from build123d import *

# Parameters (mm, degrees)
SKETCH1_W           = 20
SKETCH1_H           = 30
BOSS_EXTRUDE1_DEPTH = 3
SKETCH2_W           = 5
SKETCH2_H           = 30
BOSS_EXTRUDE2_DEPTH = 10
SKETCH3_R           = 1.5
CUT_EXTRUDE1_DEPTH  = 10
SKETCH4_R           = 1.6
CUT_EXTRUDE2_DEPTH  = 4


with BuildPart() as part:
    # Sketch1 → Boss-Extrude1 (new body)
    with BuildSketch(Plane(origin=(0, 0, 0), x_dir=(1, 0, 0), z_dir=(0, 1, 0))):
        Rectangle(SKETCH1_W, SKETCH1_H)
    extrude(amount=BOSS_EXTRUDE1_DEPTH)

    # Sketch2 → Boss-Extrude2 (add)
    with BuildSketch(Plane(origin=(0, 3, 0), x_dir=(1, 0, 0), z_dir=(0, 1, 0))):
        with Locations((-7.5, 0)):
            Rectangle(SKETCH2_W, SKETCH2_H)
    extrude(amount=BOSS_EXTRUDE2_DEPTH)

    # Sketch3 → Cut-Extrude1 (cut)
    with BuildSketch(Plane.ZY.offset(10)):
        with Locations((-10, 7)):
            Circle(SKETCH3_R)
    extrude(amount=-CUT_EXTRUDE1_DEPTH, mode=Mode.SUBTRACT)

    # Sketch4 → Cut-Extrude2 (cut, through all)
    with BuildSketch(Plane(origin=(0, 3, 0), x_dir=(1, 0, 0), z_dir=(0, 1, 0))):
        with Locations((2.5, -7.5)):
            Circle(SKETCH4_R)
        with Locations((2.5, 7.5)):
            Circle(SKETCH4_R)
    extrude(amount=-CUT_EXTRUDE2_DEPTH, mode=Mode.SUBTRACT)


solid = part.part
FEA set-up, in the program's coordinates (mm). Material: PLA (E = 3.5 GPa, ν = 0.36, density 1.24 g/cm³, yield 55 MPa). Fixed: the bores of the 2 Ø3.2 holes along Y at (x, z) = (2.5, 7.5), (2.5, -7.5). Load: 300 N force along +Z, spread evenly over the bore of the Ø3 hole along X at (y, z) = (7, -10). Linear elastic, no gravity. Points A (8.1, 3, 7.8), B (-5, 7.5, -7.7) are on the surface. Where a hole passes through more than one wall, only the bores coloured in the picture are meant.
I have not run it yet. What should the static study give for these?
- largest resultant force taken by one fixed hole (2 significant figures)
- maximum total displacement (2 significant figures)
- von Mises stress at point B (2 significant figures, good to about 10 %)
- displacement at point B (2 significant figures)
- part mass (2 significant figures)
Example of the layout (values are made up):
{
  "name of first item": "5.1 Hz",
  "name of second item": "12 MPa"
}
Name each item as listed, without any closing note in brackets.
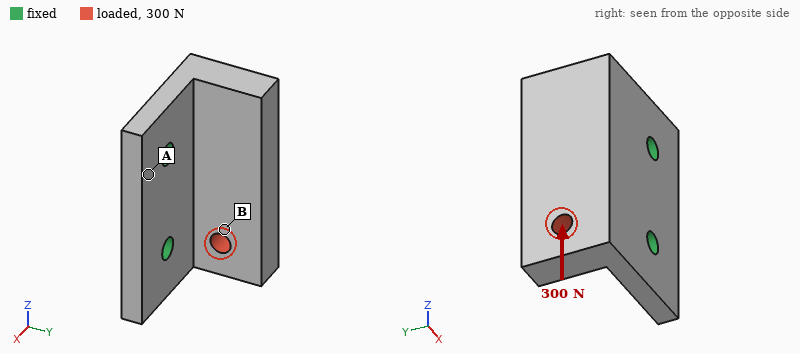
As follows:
{
  "largest resultant force taken by one fixed hole": "240 N",
  "maximum total displacement": "0.23 mm",
  "von Mises stress at point B": "11 MPa",
  "displacement at point B": "0.13 mm",
  "part mass": "4.0 g"
}
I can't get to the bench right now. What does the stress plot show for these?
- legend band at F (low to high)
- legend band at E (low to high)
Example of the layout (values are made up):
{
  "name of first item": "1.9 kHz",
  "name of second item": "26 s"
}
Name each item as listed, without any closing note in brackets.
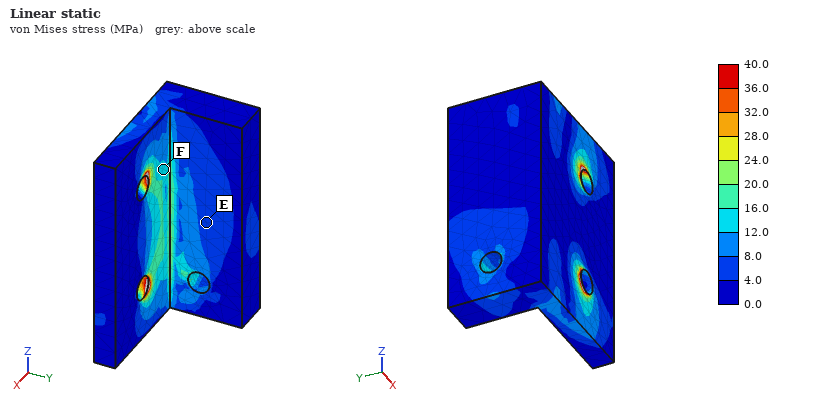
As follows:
{
  "legend band at F": "12.0 to 16.0 MPa",
  "legend band at E": "4.0 to 8.0 MPa"
}
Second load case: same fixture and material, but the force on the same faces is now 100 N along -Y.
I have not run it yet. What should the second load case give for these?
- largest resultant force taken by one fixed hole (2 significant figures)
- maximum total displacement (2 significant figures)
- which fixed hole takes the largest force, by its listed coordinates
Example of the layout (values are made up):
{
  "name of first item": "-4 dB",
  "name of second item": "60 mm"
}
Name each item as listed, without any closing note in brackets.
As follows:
{
  "largest resultant force taken by one fixed hole": "100 N",
  "maximum total displacement": "0.40 mm",
  "which fixed hole takes the largest force, by its listed coordinates": "(2.5, -7.5)"
}
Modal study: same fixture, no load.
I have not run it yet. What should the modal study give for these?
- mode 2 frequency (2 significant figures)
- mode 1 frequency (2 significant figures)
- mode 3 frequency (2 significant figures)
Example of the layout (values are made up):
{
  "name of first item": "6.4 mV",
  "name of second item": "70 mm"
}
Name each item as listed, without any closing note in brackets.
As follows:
{
  "mode 2 frequency": "3600 Hz",
  "mode 1 frequency": "2000 Hz",
  "mode 3 frequency": "6800 Hz"
}
